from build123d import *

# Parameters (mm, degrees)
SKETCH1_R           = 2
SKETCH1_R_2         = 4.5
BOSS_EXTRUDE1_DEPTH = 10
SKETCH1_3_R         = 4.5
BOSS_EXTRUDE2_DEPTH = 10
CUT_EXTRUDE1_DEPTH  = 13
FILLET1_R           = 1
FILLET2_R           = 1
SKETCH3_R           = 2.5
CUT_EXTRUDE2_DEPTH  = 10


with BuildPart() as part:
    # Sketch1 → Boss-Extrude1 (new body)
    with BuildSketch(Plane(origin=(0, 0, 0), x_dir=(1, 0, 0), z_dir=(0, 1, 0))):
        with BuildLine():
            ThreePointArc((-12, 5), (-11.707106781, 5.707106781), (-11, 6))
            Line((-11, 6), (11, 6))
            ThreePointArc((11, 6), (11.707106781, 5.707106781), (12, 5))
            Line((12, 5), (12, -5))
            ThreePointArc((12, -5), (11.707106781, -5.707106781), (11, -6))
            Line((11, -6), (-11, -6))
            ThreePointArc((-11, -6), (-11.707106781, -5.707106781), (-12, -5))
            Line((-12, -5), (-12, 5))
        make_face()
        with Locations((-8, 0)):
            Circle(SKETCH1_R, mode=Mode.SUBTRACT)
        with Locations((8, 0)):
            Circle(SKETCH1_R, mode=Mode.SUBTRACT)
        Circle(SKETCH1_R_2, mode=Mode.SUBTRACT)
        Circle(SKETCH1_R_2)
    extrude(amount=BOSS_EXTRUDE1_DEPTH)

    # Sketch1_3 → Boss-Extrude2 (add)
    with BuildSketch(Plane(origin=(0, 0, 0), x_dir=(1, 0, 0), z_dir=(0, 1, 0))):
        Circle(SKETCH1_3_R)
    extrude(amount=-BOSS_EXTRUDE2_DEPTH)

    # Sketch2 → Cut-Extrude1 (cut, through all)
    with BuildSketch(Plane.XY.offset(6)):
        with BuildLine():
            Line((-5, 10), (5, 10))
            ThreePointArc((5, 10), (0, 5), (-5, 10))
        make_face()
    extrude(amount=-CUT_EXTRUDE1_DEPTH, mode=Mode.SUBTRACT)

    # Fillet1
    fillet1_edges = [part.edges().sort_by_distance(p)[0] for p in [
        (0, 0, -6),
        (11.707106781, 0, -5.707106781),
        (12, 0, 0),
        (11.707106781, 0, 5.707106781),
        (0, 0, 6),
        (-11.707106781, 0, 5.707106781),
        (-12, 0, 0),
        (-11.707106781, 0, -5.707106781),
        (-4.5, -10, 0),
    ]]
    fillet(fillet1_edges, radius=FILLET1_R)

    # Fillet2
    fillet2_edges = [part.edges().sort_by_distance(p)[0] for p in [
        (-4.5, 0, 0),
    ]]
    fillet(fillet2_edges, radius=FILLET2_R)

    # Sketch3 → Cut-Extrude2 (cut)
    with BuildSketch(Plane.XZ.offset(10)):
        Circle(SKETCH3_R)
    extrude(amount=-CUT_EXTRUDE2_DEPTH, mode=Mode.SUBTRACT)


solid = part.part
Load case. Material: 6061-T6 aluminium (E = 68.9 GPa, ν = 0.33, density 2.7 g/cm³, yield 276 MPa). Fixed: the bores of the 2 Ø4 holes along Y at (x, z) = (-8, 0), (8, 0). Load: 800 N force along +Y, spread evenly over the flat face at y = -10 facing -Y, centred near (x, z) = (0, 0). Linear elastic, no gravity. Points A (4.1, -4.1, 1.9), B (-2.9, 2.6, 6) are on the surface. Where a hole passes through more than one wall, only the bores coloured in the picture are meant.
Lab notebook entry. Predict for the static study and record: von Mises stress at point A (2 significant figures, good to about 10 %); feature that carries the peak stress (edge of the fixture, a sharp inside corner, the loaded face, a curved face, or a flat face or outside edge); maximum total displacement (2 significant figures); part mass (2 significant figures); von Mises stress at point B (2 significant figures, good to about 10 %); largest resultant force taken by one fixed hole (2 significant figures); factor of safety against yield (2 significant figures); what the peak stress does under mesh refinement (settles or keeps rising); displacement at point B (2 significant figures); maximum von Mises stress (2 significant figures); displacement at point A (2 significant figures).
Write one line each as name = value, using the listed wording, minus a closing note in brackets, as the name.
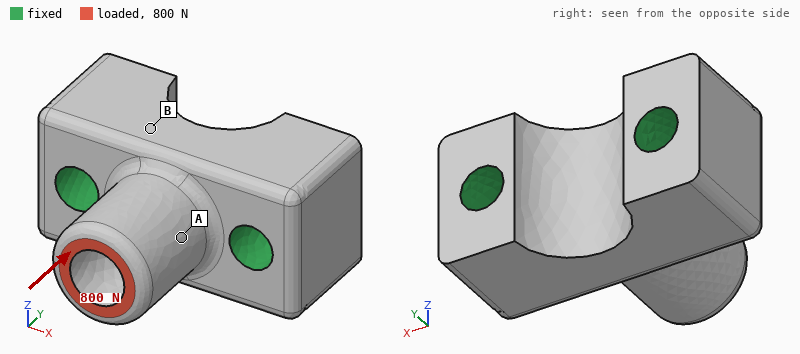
von Mises stress at point A = 18 MPa
feature that carries the peak stress = a curved face
maximum total displacement = 4.8 µm
part mass = 7.0 g
von Mises stress at point B = 7.2 MPa
largest resultant force taken by one fixed hole = 430 N
factor of safety against yield = 6.0
what the peak stress does under mesh refinement = settles
displacement at point B = 0.94 µm
maximum von Mises stress = 46 MPa
displacement at point A = 2.3 µm
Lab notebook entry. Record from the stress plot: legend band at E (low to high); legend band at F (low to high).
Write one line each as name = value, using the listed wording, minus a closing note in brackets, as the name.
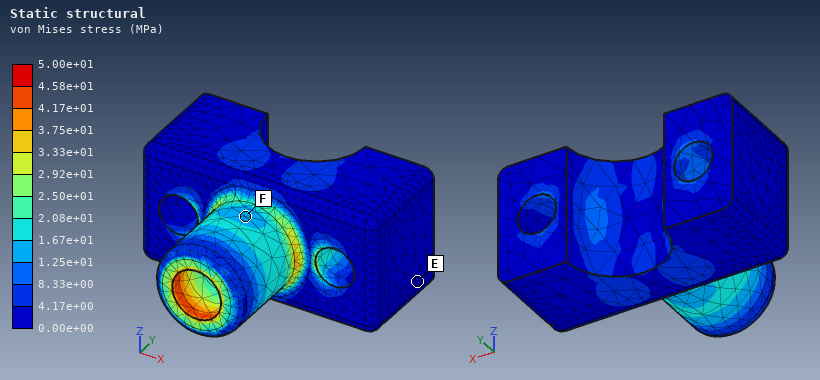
legend band at E = 0.00e+00 to 4.17e+00 MPa
legend band at F = 1.25e+01 to 1.67e+01 MPa
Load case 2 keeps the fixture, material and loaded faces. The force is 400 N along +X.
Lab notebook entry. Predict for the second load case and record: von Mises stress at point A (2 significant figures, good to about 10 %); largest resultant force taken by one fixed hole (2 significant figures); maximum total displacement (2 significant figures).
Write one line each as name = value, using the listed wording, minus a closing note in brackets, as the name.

von Mises stress at point A = 34 MPa
largest resultant force taken by one fixed hole = 460 N
maximum total displacement = 17 µm
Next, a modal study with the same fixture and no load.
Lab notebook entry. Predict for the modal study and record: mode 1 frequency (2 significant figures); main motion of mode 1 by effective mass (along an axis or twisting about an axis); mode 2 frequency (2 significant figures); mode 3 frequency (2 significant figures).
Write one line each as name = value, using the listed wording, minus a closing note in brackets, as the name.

mode 1 frequency = 33 kHz
main motion of mode 1 by effective mass = along Z
mode 2 frequency = 41 kHz
mode 3 frequency = 71 kHz
